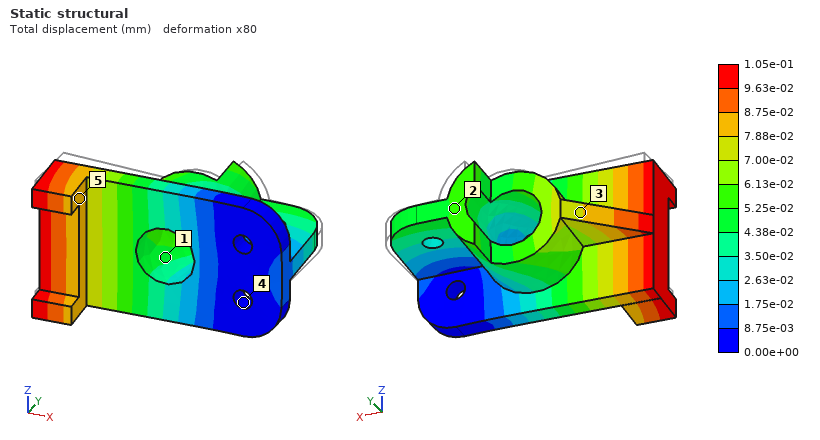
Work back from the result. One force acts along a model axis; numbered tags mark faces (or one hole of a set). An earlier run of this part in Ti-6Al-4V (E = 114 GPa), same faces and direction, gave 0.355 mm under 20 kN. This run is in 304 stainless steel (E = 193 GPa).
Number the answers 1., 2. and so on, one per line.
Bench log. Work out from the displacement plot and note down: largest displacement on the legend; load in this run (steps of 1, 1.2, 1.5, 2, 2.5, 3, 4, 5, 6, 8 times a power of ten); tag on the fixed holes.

1. 1.05e-01 mm
2. 10 kN
3. 4
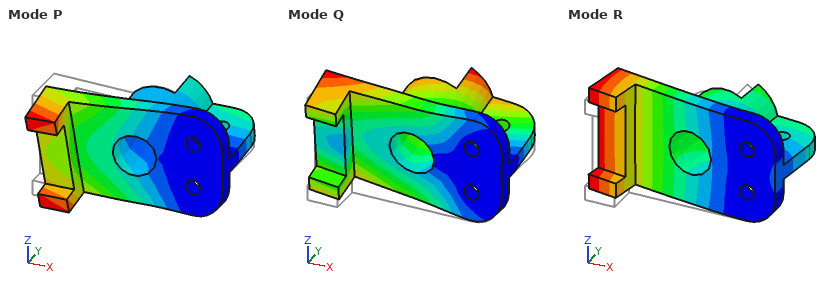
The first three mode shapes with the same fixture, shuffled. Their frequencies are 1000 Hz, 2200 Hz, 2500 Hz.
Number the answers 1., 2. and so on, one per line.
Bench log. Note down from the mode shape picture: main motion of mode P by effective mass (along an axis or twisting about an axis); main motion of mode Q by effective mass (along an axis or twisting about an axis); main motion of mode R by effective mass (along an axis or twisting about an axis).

1. along Z
2. along Z
3. along Y
